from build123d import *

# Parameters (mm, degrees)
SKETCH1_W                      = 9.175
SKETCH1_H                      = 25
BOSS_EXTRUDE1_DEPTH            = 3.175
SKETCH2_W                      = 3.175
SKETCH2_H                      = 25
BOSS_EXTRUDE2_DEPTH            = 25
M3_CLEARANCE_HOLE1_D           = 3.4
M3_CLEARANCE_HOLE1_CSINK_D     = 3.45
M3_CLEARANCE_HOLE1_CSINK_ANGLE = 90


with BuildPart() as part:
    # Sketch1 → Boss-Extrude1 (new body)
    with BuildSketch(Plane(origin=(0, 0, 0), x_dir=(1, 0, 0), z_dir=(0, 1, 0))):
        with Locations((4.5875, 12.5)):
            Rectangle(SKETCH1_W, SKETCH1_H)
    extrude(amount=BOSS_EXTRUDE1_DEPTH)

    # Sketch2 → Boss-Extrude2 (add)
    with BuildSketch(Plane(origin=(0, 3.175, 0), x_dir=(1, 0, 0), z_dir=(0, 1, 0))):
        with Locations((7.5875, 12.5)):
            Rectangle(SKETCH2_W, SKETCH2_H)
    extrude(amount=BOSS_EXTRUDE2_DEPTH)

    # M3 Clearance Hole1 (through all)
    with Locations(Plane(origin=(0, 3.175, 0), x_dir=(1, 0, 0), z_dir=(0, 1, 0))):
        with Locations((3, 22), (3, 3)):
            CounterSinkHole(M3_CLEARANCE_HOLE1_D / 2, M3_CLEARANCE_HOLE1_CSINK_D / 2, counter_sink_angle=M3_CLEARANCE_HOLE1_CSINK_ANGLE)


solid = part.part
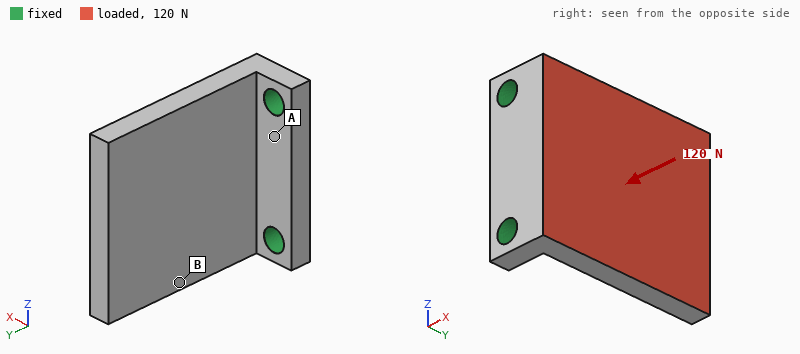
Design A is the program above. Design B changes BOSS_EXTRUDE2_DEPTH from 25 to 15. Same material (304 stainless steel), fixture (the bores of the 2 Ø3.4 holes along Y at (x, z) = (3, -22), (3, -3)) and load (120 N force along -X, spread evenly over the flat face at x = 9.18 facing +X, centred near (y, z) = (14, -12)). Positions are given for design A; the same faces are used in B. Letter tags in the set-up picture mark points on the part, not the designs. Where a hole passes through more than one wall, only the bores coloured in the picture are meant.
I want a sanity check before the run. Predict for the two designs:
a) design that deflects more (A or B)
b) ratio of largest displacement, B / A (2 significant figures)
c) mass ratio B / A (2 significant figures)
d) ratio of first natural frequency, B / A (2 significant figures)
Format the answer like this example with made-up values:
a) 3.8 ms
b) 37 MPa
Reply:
a) A
b) 0.29
c) 0.70
d) 2.3
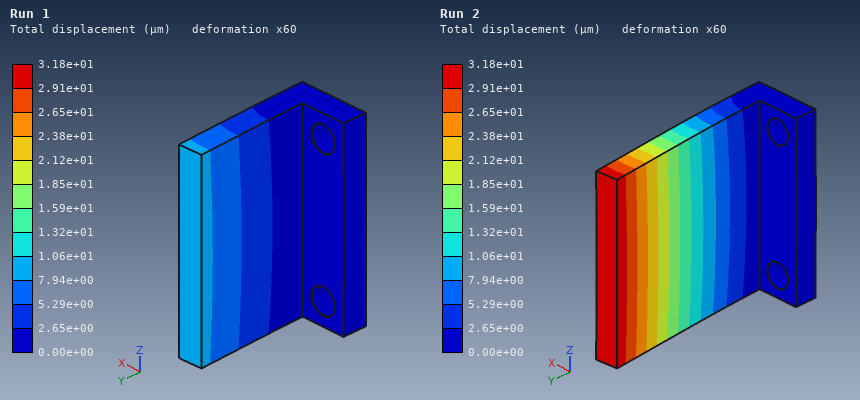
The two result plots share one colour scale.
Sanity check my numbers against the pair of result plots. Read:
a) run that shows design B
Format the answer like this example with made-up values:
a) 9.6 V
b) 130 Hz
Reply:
a) Run 1
